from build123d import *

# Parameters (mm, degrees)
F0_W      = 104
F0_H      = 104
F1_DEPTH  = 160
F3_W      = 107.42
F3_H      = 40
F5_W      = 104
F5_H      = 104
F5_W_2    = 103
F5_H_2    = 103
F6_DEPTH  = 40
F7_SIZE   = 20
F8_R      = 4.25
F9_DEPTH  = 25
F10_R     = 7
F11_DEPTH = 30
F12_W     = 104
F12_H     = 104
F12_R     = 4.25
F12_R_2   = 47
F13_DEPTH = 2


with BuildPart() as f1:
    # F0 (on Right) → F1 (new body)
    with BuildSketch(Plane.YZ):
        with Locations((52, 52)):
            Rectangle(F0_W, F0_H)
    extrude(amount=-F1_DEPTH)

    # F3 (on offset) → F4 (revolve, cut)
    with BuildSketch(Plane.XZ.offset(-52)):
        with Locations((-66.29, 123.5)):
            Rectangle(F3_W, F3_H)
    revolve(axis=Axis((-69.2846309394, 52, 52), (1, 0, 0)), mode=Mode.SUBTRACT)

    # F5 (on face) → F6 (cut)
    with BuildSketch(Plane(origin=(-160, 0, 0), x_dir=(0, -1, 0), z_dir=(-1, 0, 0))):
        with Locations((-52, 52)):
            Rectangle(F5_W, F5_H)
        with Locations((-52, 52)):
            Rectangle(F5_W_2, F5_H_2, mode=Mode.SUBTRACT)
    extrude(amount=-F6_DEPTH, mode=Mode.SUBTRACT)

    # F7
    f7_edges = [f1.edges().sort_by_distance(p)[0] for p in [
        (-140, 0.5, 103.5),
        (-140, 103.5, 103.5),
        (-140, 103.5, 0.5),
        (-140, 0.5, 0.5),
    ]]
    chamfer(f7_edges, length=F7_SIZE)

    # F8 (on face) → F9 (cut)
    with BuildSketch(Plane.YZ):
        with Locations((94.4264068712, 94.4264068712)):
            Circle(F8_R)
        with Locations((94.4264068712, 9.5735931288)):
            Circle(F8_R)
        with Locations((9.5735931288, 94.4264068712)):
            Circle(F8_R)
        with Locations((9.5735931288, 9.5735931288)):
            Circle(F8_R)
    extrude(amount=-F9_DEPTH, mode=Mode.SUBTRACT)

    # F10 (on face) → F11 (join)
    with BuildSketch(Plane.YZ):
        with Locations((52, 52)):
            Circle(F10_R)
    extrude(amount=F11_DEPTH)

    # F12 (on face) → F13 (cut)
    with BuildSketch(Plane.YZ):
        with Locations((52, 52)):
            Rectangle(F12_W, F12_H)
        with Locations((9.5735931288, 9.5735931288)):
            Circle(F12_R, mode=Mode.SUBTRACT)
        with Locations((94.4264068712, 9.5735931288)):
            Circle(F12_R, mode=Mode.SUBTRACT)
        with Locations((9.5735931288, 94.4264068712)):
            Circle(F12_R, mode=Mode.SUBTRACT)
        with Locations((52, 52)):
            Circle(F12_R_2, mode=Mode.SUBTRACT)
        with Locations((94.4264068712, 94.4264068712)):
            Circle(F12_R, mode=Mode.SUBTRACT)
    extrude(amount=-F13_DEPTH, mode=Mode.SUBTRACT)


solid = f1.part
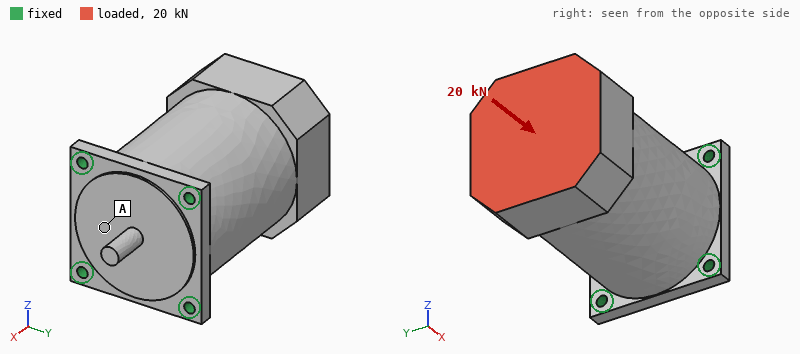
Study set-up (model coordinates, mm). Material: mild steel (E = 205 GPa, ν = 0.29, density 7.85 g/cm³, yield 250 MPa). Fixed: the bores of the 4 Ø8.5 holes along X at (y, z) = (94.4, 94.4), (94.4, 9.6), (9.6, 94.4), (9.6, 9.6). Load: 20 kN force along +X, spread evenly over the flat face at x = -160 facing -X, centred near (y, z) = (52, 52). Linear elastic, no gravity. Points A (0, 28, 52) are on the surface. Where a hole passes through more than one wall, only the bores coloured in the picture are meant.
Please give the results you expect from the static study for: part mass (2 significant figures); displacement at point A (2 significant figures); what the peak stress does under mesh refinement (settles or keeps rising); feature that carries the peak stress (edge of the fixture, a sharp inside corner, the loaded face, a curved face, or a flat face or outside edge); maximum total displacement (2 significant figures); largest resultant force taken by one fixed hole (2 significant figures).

11 kg
5.2 µm
keeps rising
edge of the fixture
6.6 µm
5.3 kN
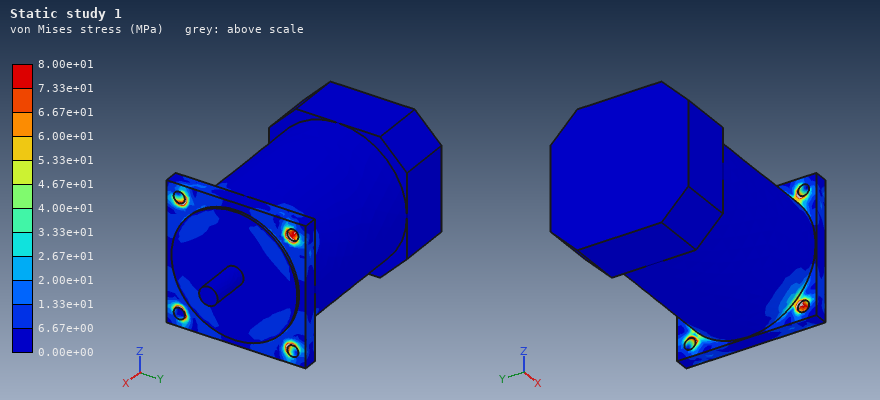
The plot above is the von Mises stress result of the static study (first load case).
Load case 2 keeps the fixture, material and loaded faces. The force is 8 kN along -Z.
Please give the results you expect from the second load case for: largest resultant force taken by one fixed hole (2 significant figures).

8.3 kN
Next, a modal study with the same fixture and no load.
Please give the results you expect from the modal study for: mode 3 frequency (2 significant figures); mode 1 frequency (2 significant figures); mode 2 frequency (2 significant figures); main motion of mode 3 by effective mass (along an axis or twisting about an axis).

2900 Hz
1200 Hz
1200 Hz
along X
